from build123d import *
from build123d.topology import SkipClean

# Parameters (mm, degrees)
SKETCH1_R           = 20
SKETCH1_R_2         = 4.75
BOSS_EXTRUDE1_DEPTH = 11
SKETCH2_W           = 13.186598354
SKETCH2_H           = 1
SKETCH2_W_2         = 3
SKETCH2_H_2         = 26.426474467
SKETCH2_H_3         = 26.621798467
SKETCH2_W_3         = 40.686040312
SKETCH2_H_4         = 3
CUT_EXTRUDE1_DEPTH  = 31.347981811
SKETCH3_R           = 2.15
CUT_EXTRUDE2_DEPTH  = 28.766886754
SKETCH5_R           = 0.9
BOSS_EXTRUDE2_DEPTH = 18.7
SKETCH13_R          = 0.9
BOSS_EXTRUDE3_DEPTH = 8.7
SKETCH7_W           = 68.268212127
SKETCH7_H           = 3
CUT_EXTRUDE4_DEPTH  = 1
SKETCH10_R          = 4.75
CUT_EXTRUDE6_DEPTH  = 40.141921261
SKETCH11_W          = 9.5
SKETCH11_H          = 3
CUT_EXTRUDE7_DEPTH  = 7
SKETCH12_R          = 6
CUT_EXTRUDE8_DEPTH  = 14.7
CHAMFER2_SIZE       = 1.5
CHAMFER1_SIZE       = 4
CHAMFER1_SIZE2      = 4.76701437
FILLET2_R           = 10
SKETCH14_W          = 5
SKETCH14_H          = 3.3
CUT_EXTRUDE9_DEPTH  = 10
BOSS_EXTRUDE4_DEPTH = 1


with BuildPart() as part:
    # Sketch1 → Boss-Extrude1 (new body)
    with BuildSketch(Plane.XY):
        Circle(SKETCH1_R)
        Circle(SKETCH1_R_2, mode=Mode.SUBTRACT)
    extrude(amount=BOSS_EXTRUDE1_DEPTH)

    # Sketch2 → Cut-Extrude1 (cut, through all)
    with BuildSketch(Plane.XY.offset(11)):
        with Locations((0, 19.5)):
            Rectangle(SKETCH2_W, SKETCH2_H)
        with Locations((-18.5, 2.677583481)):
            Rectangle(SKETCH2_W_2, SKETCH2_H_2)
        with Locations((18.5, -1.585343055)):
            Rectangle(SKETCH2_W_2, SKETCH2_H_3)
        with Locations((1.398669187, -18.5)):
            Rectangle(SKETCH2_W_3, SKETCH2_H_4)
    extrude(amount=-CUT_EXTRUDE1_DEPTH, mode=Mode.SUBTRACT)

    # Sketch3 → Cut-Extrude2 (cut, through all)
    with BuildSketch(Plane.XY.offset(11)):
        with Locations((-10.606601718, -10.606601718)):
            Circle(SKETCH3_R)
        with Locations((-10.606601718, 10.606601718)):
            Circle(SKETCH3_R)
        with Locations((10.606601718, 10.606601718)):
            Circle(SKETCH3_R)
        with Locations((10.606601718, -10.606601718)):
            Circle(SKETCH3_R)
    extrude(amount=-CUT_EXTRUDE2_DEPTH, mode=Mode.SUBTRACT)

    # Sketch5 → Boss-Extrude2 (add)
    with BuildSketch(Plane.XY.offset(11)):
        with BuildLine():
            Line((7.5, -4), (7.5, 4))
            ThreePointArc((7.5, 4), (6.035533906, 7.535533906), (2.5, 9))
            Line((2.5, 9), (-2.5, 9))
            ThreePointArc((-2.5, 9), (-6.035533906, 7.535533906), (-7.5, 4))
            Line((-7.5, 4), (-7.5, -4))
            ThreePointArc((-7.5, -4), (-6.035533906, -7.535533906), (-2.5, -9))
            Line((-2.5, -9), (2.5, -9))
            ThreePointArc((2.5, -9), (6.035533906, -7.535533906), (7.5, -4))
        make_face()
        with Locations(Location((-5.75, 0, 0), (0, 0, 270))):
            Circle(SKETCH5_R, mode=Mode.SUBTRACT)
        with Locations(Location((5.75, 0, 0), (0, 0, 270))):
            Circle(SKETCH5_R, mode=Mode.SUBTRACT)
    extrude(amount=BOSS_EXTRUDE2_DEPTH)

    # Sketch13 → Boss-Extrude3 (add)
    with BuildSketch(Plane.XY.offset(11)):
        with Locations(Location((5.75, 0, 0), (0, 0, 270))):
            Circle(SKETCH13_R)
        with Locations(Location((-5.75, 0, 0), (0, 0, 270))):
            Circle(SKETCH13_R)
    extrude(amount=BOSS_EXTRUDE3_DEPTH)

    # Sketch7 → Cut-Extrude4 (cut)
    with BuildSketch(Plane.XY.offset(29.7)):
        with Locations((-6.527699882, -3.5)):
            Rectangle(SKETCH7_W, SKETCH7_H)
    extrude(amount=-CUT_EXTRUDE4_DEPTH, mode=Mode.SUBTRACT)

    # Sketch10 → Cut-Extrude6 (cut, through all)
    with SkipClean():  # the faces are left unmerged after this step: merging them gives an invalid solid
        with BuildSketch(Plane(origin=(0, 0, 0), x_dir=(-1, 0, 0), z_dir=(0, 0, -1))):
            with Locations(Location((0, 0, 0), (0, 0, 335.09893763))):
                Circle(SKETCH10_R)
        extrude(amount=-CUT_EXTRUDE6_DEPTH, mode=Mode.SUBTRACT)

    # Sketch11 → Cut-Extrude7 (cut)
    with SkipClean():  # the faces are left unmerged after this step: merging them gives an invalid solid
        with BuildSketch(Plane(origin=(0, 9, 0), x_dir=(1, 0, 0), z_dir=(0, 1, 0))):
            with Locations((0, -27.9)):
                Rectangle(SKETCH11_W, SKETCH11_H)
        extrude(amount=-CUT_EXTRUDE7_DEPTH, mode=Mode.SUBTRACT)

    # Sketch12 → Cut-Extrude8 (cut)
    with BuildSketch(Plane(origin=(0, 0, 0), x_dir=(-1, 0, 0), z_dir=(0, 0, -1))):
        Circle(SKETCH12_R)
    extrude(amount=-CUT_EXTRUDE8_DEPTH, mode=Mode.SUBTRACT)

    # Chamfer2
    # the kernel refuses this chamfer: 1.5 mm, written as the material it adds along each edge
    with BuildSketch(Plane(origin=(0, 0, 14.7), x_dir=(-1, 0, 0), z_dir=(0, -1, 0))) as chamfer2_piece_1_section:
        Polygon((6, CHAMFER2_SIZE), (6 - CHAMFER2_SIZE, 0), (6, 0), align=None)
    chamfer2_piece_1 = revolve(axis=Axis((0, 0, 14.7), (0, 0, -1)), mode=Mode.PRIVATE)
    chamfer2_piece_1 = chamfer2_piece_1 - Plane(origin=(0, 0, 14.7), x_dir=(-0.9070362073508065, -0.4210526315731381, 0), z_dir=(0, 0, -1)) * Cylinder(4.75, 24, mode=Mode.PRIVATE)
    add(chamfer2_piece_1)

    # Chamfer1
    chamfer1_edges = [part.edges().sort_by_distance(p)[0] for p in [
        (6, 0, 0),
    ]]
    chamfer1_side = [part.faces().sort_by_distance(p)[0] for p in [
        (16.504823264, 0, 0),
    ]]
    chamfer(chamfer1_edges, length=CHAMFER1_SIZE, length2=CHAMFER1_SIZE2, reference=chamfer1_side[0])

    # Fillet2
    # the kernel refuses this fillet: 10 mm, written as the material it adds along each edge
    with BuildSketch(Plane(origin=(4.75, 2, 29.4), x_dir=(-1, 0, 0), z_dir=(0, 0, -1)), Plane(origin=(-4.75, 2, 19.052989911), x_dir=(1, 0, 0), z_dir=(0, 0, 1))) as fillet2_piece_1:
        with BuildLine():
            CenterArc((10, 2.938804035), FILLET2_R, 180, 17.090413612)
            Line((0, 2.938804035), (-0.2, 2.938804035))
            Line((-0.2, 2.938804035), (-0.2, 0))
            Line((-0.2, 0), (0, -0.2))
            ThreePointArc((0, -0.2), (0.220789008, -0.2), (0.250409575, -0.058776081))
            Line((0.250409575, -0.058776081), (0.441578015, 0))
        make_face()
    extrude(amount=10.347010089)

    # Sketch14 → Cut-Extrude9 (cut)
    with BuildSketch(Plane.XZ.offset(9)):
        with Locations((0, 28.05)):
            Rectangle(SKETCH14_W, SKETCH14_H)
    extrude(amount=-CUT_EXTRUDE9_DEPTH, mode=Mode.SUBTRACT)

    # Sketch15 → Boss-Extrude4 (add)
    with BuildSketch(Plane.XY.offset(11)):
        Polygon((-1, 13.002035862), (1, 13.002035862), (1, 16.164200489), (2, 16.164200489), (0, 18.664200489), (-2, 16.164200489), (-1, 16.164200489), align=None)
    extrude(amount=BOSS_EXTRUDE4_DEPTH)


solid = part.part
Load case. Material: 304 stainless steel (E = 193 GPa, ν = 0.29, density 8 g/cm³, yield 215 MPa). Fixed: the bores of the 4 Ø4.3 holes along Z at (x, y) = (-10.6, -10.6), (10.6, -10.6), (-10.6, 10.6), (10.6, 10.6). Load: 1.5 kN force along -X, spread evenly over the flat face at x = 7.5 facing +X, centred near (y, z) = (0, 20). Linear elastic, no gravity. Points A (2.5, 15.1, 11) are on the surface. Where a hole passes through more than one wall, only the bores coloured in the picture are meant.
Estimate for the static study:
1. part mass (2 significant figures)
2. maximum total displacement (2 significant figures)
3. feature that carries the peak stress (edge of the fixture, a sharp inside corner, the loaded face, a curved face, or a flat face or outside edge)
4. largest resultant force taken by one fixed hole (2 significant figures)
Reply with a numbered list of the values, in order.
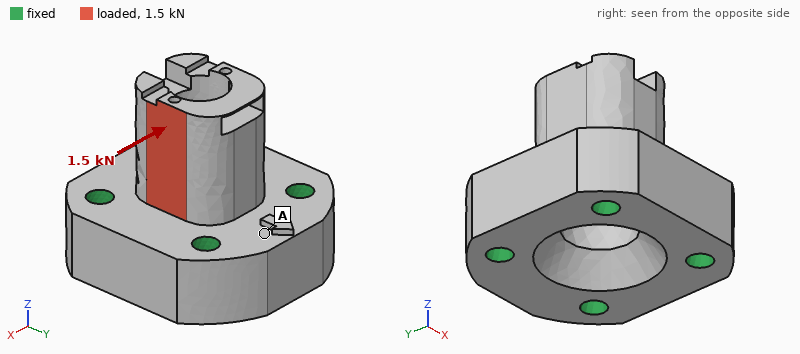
1. 100 g
2. 10 µm
3. a curved face
4. 680 N
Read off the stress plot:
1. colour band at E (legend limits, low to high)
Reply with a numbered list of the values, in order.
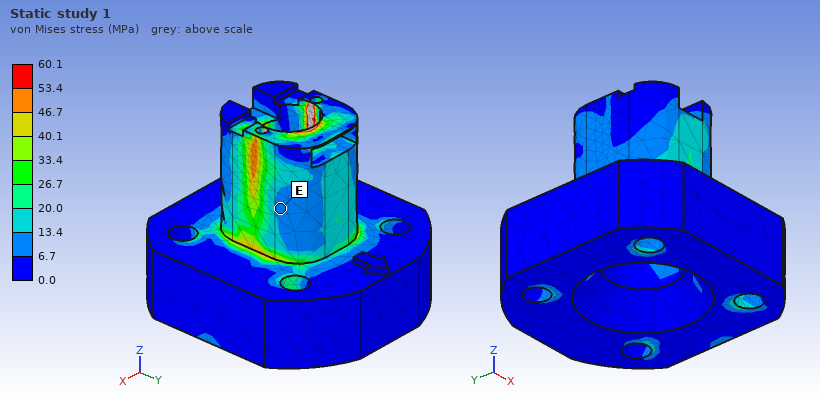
1. 6.7 to 13.4 MPa
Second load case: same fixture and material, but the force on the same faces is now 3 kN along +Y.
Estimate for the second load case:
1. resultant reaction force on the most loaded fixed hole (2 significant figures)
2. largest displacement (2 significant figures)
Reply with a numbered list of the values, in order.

1. 1.5 kN
2. 15 µm
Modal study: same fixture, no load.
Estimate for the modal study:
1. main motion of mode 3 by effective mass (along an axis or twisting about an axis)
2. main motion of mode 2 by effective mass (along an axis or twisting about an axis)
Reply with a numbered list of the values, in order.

1. along Y
2. along X
